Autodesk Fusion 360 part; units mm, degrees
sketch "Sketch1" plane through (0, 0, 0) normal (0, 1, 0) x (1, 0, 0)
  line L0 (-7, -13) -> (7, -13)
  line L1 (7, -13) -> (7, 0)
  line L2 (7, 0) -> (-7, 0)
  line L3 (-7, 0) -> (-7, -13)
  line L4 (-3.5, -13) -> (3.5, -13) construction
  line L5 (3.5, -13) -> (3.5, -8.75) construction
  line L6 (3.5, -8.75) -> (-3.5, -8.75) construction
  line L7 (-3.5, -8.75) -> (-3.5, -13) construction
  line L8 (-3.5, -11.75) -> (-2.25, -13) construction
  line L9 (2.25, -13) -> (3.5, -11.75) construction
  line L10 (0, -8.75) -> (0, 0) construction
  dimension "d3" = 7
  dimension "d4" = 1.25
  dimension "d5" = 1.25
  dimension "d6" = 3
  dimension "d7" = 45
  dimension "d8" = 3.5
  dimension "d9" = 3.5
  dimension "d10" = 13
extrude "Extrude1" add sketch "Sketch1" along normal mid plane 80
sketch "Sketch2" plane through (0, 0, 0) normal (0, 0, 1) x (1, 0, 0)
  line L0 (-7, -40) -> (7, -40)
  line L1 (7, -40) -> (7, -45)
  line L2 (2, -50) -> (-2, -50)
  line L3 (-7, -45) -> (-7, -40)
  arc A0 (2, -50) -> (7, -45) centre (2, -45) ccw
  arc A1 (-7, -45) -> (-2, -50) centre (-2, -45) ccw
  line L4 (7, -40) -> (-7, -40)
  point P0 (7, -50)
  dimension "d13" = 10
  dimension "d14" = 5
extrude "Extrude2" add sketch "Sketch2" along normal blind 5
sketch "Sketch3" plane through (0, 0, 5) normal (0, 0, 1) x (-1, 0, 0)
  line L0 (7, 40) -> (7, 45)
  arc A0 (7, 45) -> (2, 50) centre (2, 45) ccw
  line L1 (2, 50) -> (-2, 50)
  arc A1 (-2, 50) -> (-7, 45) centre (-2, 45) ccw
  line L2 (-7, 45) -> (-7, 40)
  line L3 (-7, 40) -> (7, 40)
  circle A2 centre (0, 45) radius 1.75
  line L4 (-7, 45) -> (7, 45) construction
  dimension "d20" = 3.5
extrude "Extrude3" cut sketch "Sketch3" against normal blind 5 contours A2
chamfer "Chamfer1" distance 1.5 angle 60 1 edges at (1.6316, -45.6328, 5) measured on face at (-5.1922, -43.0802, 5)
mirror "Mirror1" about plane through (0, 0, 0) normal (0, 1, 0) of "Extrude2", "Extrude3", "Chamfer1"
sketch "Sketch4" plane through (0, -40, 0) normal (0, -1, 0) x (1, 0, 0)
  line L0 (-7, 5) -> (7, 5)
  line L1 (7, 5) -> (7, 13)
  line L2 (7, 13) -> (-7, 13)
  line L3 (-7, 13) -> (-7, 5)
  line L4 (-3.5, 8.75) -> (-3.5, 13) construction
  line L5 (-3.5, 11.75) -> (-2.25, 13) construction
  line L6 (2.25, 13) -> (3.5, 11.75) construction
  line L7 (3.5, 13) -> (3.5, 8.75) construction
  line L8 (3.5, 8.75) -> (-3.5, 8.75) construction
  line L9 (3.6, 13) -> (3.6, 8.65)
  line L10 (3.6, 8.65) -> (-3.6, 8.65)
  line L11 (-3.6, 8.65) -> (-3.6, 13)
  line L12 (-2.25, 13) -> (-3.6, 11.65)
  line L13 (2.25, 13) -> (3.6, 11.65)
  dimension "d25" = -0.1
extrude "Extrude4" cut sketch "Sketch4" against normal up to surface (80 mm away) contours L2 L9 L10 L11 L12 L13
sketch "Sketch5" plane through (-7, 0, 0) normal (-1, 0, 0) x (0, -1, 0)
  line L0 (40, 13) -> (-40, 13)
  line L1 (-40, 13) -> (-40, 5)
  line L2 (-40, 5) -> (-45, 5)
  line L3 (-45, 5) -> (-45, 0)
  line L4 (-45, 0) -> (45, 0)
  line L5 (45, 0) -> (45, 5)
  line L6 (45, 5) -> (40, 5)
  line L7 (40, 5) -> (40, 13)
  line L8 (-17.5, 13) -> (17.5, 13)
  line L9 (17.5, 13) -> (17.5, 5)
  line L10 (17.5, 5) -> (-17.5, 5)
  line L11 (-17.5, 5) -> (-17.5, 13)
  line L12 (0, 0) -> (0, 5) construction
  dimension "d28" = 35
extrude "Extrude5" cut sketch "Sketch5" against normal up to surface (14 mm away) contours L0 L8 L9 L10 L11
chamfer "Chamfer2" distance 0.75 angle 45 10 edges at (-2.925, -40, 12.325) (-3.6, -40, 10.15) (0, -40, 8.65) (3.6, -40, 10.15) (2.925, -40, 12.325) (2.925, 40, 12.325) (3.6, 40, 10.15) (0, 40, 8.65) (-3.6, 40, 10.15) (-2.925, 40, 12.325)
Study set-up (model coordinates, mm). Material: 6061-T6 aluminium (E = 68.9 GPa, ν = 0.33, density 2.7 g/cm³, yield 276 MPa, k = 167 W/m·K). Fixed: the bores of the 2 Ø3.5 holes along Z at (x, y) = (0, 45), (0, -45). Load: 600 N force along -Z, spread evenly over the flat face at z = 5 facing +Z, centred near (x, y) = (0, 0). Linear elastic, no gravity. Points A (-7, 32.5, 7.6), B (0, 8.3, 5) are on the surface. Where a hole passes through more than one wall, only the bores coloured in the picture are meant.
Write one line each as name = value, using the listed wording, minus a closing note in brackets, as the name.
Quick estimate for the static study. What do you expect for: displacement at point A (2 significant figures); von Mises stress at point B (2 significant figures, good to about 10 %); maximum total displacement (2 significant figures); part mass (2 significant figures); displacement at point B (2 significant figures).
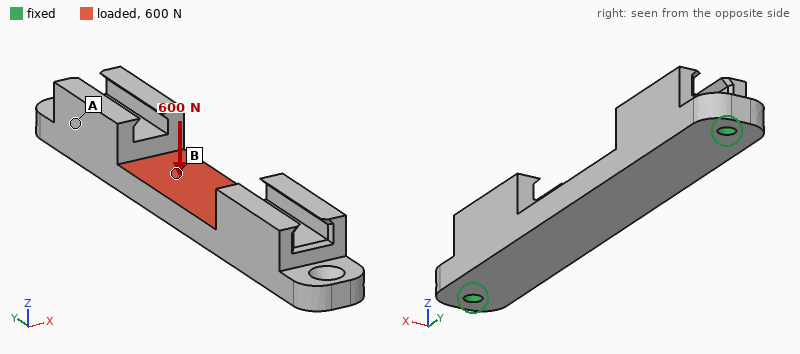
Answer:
displacement at point A = 0.080 mm
von Mises stress at point B = 76 MPa
maximum total displacement = 0.25 mm
part mass = 28 g
displacement at point B = 0.23 mm
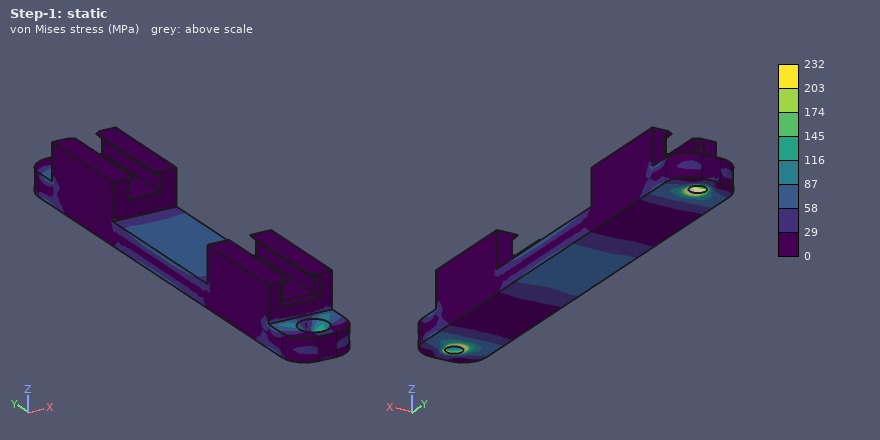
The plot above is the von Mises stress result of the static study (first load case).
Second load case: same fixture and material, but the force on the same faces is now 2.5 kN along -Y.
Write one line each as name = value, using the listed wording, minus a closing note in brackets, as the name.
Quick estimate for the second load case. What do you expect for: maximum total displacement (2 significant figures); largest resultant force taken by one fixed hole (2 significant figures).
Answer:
maximum total displacement = 13 µm
largest resultant force taken by one fixed hole = 1.3 kN
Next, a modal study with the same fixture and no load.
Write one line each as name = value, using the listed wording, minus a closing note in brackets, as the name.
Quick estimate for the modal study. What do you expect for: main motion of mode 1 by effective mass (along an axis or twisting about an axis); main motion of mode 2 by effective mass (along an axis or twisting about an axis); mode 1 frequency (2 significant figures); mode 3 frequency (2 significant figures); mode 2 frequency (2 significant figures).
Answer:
main motion of mode 1 by effective mass = along Z
main motion of mode 2 by effective mass = along X
mode 1 frequency = 2400 Hz
mode 3 frequency = 6800 Hz
mode 2 frequency = 4600 Hz
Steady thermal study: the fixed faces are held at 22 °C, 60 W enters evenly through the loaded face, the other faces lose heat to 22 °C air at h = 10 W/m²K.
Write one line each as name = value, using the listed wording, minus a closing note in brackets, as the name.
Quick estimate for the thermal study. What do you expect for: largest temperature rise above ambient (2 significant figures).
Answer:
largest temperature rise above ambient = 74 K
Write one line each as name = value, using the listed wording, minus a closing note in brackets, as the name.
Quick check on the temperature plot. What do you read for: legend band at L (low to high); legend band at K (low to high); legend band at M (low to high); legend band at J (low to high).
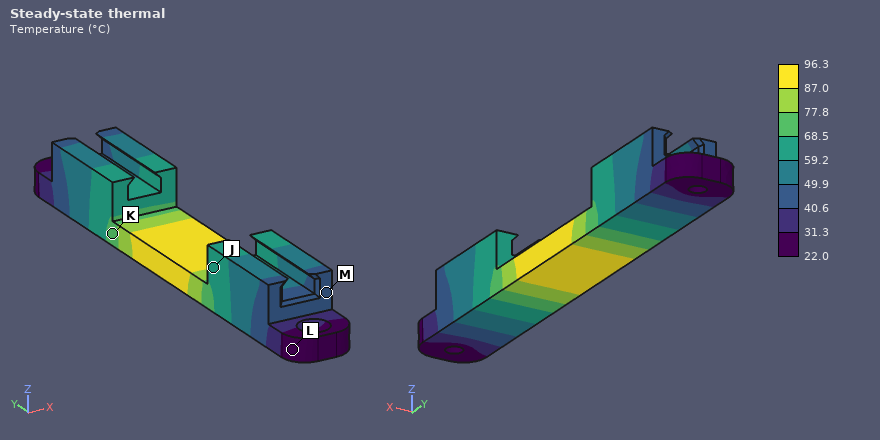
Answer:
legend band at L = 22.0 to 31.3 °C
legend band at K = 68.5 to 77.8 °C
legend band at M = 40.6 to 49.9 °C
legend band at J = 59.2 to 68.5 °C
